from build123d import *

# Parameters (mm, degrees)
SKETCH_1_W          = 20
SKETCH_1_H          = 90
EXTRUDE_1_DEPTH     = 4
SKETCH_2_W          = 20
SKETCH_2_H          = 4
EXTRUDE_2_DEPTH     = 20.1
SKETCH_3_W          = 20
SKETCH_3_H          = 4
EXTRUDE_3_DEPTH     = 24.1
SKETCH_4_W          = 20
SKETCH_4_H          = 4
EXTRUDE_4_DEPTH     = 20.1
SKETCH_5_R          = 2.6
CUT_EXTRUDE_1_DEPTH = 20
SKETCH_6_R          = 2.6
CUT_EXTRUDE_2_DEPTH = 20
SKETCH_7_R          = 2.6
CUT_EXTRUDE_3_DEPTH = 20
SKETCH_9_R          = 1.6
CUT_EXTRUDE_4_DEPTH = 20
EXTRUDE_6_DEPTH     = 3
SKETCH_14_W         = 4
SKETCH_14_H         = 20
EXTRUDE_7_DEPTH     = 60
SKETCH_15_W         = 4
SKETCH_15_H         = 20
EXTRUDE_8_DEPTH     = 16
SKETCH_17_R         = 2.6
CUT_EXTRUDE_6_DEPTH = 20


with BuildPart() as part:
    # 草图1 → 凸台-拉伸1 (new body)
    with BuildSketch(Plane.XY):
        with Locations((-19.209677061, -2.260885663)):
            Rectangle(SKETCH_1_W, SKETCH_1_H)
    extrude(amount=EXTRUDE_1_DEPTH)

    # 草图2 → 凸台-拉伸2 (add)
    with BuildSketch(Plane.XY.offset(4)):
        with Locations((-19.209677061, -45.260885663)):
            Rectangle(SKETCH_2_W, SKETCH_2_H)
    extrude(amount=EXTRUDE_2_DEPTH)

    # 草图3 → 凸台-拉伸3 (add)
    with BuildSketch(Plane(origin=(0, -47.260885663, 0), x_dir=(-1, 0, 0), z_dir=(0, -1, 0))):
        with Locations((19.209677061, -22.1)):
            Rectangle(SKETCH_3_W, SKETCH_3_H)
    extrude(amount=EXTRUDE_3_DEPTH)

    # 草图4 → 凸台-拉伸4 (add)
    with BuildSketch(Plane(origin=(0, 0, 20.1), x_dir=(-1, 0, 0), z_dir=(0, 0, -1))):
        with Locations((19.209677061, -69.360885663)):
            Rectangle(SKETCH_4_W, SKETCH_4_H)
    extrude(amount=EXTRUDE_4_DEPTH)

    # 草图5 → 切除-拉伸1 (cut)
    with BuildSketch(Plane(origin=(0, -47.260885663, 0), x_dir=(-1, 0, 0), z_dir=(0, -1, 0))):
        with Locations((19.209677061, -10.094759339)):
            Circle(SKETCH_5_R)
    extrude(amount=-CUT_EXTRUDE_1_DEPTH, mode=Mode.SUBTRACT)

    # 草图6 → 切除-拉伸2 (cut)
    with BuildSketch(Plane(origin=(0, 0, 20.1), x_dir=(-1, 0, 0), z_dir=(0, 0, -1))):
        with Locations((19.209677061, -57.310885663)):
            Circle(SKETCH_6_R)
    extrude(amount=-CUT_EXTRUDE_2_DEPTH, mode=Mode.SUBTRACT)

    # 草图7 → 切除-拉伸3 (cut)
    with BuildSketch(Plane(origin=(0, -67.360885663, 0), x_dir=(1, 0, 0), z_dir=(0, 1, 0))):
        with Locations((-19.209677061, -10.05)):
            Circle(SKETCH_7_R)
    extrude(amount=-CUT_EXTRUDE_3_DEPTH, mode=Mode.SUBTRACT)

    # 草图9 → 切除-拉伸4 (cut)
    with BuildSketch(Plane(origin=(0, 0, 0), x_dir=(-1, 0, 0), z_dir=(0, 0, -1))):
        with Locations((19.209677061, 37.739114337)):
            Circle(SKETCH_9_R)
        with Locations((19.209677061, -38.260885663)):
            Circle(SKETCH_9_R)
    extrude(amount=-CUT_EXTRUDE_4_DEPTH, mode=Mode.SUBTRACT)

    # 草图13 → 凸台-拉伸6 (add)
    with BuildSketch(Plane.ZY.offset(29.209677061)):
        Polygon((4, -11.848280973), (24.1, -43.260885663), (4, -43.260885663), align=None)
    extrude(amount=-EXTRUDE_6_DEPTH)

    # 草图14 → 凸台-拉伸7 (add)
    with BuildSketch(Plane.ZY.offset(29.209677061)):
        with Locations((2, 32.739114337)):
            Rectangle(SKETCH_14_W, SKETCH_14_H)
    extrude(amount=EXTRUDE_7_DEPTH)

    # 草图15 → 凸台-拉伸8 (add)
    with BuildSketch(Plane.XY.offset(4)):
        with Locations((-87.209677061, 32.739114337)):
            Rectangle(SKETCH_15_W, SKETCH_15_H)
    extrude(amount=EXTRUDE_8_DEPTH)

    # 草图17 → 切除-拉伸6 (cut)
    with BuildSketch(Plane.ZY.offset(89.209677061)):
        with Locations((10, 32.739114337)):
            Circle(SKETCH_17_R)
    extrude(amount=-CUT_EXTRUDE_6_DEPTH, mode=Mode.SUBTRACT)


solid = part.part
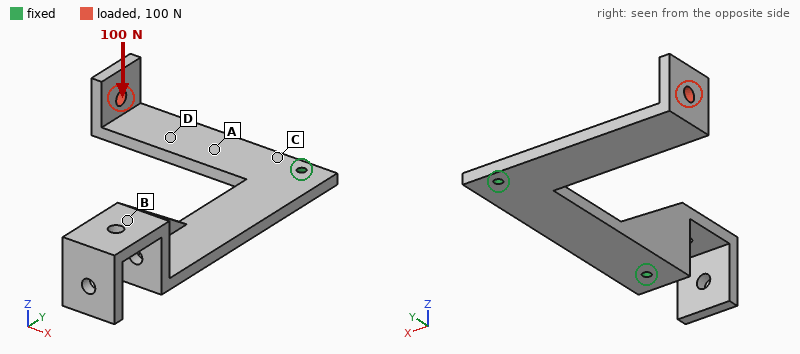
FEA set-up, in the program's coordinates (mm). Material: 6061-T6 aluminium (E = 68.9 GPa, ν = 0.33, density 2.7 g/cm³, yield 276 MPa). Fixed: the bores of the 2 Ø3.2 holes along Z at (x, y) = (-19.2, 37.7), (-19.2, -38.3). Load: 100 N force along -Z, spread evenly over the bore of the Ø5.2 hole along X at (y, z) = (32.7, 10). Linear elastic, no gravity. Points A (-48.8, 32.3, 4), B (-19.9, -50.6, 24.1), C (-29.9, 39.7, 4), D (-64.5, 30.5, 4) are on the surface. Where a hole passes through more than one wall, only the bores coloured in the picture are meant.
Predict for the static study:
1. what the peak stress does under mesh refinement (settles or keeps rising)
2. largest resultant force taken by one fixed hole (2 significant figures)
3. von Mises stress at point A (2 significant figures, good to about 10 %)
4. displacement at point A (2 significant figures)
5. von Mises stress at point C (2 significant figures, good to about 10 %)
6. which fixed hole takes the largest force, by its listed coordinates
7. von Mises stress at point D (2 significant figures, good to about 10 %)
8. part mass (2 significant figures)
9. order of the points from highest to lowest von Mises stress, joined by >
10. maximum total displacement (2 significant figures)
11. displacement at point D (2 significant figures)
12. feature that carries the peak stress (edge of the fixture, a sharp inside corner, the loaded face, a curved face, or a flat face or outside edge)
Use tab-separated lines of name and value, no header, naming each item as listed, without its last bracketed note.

what the peak stress does under mesh refinement	keeps rising
largest resultant force taken by one fixed hole	110 N
von Mises stress at point A	72 MPa
displacement at point A	0.37 mm
von Mises stress at point C	110 MPa
which fixed hole takes the largest force, by its listed coordinates	(-19.2, 37.7)
von Mises stress at point D	42 MPa
part mass	51 g
order of the points from highest to lowest von Mises stress, joined by >	C > A > D > B
maximum total displacement	1.6 mm
displacement at point D	0.76 mm
feature that carries the peak stress	edge of the fixture
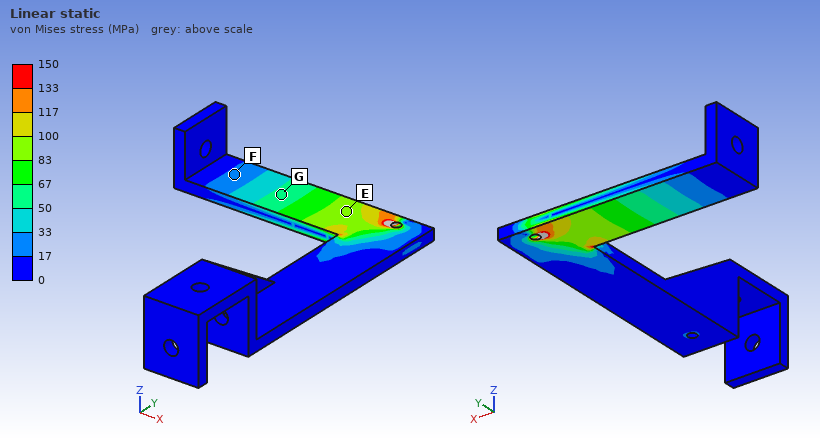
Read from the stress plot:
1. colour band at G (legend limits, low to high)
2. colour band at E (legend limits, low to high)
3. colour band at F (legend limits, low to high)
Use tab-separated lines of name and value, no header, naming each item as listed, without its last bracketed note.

colour band at G	50 to 67 MPa
colour band at E	83 to 100 MPa
colour band at F	17 to 33 MPa
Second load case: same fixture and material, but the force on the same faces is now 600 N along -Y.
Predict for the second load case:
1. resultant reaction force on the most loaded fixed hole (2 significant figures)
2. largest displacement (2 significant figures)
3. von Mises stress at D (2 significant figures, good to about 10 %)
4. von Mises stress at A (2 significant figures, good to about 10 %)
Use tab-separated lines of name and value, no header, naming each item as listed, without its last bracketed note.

resultant reaction force on the most loaded fixed hole	570 N
largest displacement	1.1 mm
von Mises stress at D	110 MPa
von Mises stress at A	110 MPa
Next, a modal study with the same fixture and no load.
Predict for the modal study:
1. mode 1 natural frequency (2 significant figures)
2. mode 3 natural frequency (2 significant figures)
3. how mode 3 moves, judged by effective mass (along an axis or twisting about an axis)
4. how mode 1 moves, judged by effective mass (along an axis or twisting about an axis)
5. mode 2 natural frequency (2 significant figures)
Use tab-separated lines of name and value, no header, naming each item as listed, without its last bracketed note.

mode 1 natural frequency	490 Hz
mode 3 natural frequency	1700 Hz
how mode 3 moves, judged by effective mass	along Y
how mode 1 moves, judged by effective mass	along Z
mode 2 natural frequency	1500 Hz
